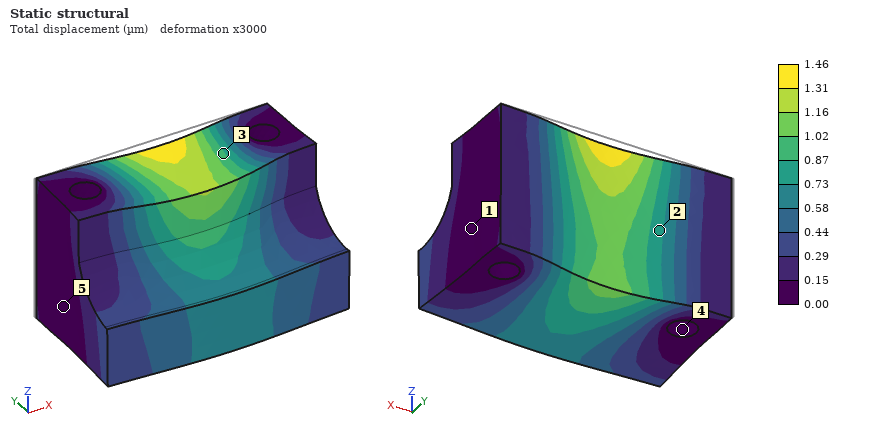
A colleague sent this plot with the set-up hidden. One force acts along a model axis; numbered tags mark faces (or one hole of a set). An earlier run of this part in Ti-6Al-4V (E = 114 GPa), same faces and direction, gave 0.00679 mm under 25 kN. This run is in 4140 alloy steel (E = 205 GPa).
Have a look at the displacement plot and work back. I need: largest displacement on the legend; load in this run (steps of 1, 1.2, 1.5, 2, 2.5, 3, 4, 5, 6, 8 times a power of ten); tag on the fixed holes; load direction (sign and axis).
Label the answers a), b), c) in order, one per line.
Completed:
a) 1.46 µm
b) 10 kN
c) 4
d) -Y
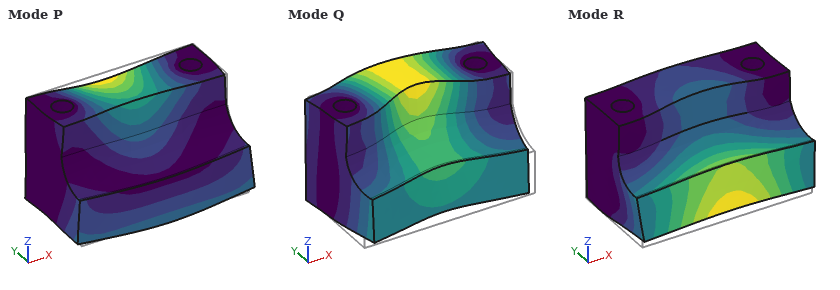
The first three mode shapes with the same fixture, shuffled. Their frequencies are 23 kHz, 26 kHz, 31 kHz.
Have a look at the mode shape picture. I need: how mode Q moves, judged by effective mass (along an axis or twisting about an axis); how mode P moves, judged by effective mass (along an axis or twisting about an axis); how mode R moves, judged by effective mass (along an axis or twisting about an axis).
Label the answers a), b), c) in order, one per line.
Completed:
a) along Y
b) along Z
c) along Z
